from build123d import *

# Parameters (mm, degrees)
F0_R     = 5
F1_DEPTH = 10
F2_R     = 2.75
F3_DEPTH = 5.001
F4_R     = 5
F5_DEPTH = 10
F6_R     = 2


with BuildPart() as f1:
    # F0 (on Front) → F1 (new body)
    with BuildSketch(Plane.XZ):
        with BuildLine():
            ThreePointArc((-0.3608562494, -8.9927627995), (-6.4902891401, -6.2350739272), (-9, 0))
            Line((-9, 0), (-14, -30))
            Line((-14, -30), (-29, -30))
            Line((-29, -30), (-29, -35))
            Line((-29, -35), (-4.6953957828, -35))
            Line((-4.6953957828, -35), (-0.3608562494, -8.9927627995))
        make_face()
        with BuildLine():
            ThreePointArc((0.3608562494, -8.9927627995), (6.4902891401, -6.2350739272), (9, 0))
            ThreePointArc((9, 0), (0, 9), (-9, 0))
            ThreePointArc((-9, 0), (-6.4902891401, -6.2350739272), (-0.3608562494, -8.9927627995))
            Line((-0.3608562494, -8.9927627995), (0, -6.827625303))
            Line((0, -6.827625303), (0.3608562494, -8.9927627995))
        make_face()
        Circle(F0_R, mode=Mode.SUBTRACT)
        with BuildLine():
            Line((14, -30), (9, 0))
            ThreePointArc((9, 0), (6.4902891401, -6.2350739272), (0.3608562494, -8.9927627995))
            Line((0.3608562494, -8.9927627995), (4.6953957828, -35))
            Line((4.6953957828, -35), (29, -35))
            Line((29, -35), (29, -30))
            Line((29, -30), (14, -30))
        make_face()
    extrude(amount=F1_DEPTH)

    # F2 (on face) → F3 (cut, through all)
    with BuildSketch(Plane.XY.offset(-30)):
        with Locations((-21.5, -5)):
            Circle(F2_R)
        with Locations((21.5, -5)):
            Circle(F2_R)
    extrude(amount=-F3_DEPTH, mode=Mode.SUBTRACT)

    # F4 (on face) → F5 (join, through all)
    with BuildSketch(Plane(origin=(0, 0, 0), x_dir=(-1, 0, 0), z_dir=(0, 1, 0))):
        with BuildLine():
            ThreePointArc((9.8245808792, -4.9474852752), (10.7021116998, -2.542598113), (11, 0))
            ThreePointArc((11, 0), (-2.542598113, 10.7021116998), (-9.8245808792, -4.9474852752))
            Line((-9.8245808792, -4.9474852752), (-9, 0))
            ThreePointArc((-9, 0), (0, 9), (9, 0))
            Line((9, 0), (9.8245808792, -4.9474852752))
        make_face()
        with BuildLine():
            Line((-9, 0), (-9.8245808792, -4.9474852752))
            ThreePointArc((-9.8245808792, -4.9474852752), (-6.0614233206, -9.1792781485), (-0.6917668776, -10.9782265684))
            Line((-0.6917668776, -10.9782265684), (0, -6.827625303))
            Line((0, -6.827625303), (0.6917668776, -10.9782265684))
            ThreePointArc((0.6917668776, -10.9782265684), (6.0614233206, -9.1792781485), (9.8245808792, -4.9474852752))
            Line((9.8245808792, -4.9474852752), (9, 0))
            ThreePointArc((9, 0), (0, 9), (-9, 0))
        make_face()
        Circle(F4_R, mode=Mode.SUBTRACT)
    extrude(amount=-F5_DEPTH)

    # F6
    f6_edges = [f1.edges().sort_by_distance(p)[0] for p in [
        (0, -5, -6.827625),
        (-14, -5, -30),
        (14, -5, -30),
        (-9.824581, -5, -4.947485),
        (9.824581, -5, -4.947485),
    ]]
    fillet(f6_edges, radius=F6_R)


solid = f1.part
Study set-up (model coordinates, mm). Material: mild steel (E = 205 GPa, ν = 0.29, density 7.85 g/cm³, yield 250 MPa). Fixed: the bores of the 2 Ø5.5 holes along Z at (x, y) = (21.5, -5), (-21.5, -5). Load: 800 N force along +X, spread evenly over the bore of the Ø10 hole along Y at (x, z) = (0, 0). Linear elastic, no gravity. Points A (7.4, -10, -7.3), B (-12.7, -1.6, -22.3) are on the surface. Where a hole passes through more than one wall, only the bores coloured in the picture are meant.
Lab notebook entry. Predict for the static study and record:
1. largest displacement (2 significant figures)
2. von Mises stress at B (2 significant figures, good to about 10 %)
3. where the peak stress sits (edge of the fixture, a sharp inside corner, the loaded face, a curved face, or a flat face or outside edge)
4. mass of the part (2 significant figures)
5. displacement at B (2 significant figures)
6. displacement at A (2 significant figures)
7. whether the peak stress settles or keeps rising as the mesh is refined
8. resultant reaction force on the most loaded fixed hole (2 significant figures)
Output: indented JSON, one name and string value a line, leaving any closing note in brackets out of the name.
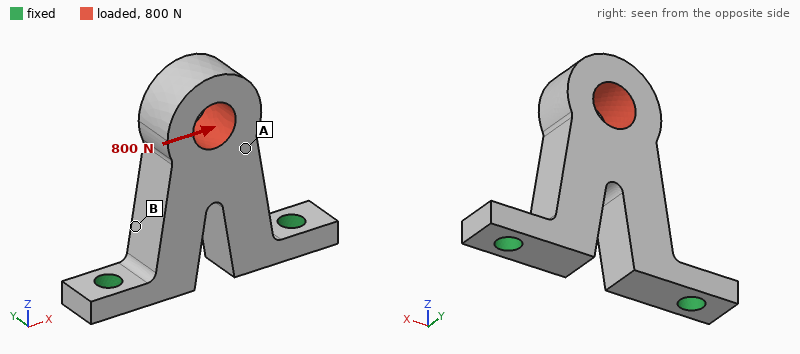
{
  "largest displacement": "16 µm",
  "von Mises stress at B": "26 MPa",
  "where the peak stress sits": "edge of the fixture",
  "mass of the part": "76 g",
  "displacement at B": "3.9 µm",
  "displacement at A": "7.8 µm",
  "whether the peak stress settles or keeps rising as the mesh is refined": "keeps rising",
  "resultant reaction force on the most loaded fixed hole": "890 N"
}
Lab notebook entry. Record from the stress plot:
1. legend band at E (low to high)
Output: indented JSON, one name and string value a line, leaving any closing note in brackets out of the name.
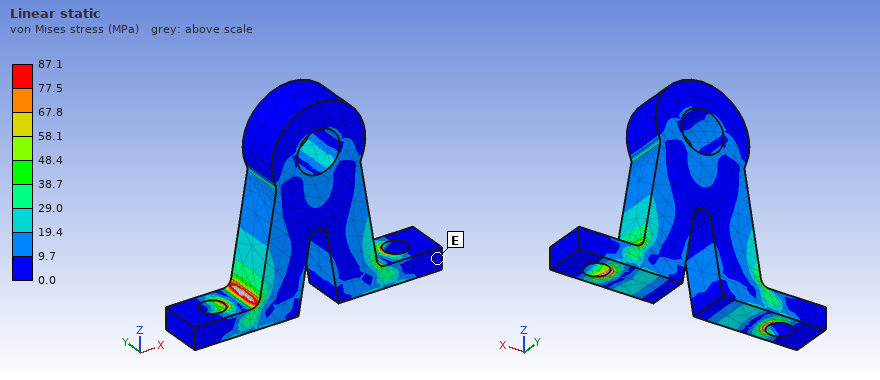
{
  "legend band at E": "0.0 to 9.7 MPa"
}
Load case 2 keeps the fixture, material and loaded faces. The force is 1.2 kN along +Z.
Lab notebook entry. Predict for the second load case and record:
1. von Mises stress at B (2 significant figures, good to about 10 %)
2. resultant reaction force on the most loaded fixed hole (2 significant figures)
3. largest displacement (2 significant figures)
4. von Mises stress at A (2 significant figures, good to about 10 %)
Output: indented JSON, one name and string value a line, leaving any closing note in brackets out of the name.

{
  "von Mises stress at B": "15 MPa",
  "resultant reaction force on the most loaded fixed hole": "690 N",
  "largest displacement": "4.3 µm",
  "von Mises stress at A": "6.9 MPa"
}
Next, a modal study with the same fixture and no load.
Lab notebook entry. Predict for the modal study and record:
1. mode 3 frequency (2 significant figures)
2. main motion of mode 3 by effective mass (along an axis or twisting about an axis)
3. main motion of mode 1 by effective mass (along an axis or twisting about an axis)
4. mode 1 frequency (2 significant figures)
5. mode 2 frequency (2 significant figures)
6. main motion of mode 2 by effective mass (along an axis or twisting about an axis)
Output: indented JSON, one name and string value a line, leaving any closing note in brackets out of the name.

{
  "mode 3 frequency": "12 kHz",
  "main motion of mode 3 by effective mass": "along Z",
  "main motion of mode 1 by effective mass": "along Y",
  "mode 1 frequency": "2200 Hz",
  "mode 2 frequency": "7600 Hz",
  "main motion of mode 2 by effective mass": "along X"
}
